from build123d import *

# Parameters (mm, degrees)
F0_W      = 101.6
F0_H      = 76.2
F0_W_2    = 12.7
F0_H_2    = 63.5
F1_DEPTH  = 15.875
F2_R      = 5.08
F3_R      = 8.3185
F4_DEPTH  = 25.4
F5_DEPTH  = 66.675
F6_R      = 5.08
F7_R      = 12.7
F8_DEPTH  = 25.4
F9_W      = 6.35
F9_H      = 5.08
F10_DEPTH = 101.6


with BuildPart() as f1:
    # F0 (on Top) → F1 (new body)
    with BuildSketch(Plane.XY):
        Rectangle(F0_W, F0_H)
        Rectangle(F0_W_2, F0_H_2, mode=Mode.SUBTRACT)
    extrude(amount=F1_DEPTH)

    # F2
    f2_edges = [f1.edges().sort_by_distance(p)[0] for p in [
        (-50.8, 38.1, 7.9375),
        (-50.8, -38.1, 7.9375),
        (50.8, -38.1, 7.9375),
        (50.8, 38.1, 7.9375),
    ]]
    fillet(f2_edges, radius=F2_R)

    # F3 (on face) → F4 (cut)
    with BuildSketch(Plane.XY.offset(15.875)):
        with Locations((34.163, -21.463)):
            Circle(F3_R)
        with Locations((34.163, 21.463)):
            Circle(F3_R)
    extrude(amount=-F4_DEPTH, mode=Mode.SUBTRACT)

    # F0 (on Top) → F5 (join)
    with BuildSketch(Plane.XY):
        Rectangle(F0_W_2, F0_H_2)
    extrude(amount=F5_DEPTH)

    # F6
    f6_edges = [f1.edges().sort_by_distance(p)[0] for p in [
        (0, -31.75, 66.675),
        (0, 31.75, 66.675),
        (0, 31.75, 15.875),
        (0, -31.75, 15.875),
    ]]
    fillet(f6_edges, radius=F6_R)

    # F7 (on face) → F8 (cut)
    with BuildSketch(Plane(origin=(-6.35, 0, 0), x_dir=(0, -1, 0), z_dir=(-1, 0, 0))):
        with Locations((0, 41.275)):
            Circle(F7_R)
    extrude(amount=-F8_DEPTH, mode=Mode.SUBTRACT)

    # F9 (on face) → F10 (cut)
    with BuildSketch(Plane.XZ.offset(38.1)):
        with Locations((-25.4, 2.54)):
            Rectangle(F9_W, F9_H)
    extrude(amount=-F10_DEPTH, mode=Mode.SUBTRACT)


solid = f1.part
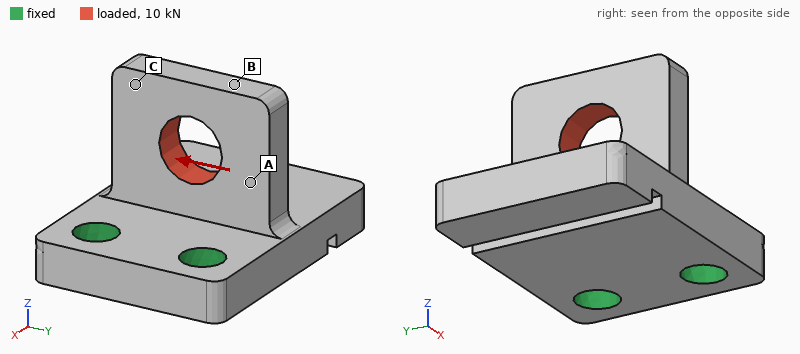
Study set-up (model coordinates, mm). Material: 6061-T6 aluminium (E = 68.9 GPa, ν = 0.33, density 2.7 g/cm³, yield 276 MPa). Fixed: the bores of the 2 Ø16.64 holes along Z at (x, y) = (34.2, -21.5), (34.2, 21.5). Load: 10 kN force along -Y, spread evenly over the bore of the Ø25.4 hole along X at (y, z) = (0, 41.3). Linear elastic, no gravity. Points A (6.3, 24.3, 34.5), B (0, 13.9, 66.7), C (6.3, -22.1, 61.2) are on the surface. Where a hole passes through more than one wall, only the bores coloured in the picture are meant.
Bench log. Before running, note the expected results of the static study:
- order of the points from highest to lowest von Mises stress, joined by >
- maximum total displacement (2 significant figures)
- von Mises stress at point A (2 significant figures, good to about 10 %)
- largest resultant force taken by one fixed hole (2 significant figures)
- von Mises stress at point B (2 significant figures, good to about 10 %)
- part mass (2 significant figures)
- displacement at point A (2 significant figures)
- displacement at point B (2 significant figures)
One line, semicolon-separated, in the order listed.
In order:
A > B > C; 0.15 mm; 35 MPa; 9.6 kN; 20 MPa; 400 g; 0.079 mm; 0.14 mm
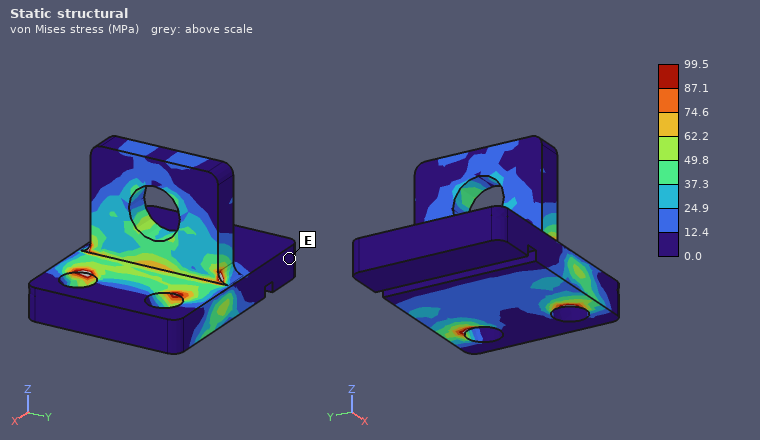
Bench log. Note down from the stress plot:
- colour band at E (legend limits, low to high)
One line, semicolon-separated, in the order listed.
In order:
0.0 to 12.4 MPa
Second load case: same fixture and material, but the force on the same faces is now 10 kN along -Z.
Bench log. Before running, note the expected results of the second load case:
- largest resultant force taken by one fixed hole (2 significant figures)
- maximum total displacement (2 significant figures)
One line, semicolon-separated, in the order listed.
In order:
5.0 kN; 0.18 mm
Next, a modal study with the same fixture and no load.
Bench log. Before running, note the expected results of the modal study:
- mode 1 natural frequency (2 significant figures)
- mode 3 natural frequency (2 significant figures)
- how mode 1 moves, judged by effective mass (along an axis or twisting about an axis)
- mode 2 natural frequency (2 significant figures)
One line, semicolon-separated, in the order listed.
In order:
1700 Hz; 3700 Hz; along Z; 3600 Hz
